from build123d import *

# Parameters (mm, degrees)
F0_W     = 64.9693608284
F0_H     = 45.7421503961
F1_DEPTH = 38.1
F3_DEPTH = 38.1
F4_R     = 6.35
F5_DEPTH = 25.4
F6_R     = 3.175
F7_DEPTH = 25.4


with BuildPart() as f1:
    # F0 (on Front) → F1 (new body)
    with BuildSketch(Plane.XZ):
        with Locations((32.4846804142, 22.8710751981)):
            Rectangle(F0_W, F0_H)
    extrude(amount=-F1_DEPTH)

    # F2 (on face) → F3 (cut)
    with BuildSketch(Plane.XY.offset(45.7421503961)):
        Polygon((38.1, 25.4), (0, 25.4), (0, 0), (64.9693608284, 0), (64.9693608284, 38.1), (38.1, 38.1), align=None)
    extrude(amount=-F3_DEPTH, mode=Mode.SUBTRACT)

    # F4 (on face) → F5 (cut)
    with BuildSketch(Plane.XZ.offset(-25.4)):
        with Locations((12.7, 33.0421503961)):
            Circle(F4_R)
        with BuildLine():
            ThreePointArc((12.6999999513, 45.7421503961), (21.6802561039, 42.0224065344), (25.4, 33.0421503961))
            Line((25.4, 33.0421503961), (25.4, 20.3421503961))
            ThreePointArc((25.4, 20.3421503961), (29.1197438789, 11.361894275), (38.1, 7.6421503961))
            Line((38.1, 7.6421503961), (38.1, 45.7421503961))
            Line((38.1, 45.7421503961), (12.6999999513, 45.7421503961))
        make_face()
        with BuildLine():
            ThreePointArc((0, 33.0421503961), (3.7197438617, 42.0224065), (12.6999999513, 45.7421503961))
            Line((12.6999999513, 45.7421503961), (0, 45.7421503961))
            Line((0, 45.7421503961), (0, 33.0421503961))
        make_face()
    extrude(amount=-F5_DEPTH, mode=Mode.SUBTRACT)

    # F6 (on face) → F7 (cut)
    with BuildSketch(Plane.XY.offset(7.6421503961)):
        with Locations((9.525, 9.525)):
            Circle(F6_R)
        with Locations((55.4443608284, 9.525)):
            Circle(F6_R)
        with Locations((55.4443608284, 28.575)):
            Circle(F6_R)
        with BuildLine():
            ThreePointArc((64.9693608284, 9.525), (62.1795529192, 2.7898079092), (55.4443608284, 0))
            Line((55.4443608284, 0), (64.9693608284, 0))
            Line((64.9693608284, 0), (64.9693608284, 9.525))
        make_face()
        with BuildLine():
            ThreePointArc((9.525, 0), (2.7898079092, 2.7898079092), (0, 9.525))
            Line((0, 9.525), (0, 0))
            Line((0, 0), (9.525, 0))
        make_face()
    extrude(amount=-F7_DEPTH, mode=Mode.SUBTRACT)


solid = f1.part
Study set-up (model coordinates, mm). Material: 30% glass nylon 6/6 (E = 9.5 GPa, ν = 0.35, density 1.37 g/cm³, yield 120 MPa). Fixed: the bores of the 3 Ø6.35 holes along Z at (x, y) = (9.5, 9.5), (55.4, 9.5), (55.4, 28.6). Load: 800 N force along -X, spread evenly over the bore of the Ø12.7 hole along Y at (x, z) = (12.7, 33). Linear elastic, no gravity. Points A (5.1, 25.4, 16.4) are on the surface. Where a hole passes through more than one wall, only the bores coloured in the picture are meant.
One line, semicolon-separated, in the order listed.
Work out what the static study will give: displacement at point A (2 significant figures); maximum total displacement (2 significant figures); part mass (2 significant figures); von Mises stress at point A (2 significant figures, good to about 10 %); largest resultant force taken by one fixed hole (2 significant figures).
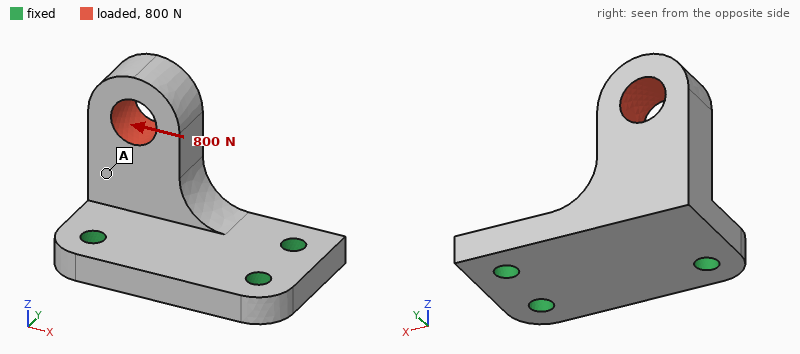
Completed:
0.19 mm; 0.46 mm; 39 g; 8.0 MPa; 600 N
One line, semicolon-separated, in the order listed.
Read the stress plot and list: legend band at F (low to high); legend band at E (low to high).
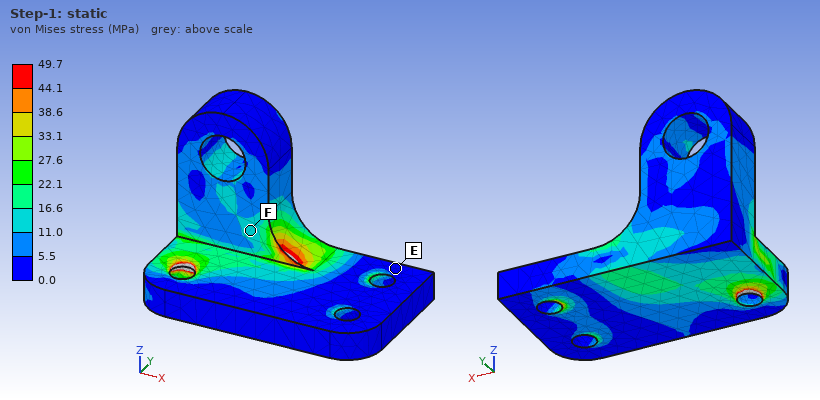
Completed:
11.0 to 16.6 MPa; 0.0 to 5.5 MPa
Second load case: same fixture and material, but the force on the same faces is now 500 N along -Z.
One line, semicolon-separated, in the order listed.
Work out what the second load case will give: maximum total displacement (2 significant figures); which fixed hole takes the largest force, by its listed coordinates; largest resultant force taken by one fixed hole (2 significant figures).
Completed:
0.30 mm; (9.5, 9.5); 410 N
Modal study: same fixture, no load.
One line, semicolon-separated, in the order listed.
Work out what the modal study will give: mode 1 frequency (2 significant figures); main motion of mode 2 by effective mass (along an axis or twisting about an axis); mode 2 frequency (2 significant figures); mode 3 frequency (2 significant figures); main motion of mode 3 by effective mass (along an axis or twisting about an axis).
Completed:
1500 Hz; along X; 2900 Hz; 4500 Hz; along Z
